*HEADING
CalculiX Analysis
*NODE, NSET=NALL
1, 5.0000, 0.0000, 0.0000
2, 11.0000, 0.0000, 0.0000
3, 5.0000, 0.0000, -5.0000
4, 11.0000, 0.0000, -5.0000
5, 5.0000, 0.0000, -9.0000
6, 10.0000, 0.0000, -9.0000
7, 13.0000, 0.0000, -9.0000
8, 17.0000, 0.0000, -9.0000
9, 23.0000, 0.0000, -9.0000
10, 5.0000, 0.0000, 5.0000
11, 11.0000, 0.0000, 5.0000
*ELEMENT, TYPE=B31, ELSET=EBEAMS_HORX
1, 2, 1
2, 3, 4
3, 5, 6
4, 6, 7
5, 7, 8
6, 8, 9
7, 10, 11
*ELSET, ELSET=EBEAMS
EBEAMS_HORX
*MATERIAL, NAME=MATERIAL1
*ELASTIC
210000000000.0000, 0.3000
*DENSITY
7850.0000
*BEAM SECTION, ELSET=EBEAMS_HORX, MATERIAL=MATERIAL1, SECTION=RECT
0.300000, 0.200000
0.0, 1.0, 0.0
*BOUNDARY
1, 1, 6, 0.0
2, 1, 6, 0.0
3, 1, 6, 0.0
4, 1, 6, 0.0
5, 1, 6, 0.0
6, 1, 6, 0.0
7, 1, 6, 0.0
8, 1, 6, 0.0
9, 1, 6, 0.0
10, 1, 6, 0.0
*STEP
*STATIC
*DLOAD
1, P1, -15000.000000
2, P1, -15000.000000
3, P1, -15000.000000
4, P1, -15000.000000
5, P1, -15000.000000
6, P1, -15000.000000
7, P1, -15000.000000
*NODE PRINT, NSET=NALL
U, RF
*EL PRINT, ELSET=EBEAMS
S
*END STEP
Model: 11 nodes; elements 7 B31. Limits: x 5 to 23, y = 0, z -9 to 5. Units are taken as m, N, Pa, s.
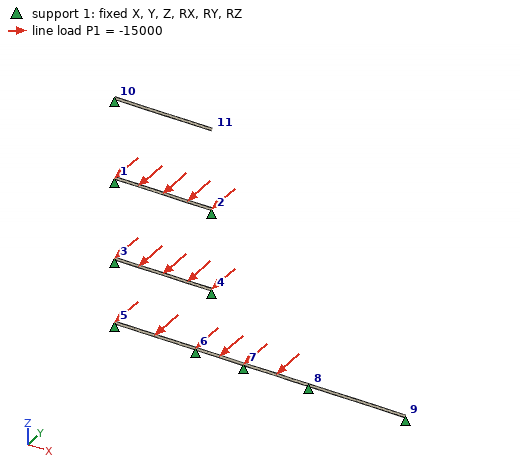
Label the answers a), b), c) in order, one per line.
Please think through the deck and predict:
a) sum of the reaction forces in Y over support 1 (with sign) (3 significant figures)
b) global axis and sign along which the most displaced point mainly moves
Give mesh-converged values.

a) 5.40e+05 N
b) -Y
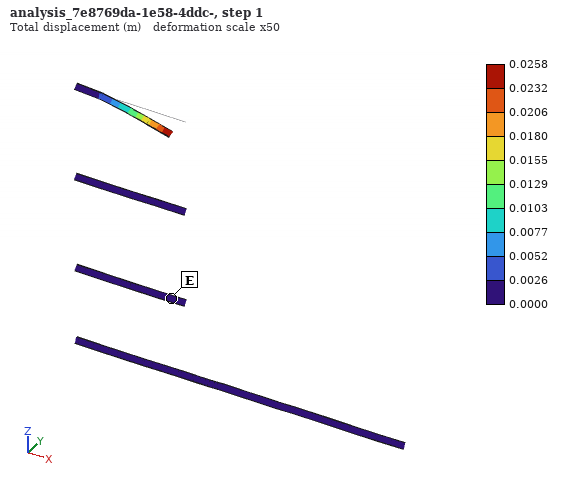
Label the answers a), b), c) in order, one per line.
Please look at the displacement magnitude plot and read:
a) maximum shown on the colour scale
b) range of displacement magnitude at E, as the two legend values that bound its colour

a) 0.0258 m
b) 0.0000 to 0.0026 m
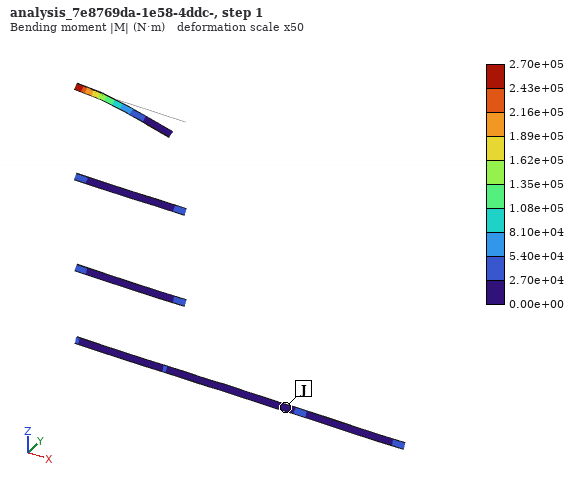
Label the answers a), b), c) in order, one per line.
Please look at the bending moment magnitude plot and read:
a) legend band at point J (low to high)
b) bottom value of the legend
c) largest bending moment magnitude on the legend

a) 0.00e+00 to 2.70e+04 N·m
b) 0.00e+00 N·m
c) 2.70e+05 N·m
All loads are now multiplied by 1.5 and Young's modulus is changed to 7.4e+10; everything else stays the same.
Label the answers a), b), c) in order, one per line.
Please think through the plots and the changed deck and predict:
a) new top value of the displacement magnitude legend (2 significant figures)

a) 0.11 m
